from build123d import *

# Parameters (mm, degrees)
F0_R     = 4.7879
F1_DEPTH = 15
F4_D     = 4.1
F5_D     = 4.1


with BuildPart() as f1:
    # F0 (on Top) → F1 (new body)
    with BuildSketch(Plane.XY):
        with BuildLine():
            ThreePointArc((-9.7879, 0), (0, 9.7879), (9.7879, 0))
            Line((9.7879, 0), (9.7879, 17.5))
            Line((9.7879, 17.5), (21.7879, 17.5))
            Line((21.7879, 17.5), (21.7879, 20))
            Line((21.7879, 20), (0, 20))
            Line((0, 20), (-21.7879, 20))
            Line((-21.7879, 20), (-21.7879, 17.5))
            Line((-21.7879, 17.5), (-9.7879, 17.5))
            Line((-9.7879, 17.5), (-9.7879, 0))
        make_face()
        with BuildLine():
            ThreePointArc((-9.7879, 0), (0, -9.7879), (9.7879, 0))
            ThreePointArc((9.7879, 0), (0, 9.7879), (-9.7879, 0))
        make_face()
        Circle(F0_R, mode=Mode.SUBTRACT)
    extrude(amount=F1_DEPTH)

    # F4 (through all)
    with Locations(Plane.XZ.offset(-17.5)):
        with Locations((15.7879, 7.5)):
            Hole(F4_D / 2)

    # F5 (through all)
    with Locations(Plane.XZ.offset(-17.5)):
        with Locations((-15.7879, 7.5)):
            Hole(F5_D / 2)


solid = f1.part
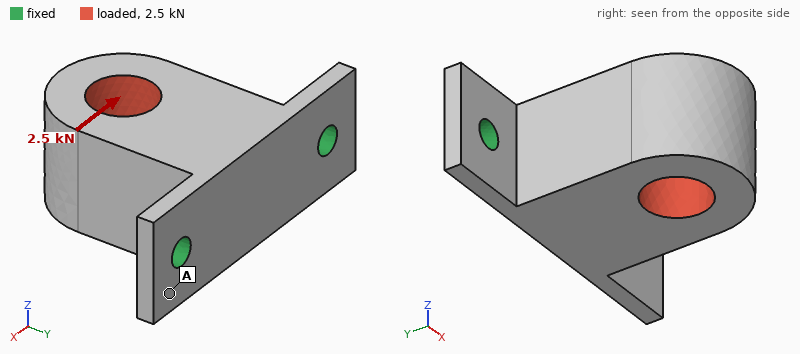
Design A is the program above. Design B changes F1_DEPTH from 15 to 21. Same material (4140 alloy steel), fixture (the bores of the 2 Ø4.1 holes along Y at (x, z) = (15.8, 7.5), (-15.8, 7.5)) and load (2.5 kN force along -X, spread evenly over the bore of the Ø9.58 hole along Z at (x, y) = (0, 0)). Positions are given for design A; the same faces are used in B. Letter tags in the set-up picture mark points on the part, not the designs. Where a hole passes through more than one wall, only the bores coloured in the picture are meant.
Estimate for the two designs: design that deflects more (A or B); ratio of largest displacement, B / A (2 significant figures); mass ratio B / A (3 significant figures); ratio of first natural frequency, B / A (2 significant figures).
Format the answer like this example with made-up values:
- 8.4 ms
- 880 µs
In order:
- A
- 0.91
- 1.40
- 0.88
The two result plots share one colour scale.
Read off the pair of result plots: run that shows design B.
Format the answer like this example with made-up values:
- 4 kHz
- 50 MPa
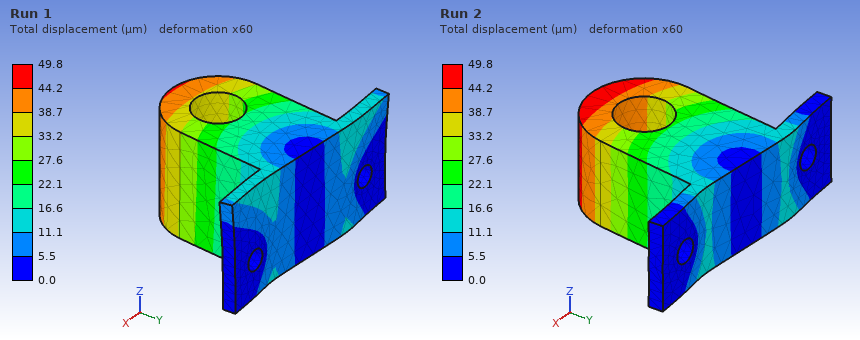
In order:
- Run 1
